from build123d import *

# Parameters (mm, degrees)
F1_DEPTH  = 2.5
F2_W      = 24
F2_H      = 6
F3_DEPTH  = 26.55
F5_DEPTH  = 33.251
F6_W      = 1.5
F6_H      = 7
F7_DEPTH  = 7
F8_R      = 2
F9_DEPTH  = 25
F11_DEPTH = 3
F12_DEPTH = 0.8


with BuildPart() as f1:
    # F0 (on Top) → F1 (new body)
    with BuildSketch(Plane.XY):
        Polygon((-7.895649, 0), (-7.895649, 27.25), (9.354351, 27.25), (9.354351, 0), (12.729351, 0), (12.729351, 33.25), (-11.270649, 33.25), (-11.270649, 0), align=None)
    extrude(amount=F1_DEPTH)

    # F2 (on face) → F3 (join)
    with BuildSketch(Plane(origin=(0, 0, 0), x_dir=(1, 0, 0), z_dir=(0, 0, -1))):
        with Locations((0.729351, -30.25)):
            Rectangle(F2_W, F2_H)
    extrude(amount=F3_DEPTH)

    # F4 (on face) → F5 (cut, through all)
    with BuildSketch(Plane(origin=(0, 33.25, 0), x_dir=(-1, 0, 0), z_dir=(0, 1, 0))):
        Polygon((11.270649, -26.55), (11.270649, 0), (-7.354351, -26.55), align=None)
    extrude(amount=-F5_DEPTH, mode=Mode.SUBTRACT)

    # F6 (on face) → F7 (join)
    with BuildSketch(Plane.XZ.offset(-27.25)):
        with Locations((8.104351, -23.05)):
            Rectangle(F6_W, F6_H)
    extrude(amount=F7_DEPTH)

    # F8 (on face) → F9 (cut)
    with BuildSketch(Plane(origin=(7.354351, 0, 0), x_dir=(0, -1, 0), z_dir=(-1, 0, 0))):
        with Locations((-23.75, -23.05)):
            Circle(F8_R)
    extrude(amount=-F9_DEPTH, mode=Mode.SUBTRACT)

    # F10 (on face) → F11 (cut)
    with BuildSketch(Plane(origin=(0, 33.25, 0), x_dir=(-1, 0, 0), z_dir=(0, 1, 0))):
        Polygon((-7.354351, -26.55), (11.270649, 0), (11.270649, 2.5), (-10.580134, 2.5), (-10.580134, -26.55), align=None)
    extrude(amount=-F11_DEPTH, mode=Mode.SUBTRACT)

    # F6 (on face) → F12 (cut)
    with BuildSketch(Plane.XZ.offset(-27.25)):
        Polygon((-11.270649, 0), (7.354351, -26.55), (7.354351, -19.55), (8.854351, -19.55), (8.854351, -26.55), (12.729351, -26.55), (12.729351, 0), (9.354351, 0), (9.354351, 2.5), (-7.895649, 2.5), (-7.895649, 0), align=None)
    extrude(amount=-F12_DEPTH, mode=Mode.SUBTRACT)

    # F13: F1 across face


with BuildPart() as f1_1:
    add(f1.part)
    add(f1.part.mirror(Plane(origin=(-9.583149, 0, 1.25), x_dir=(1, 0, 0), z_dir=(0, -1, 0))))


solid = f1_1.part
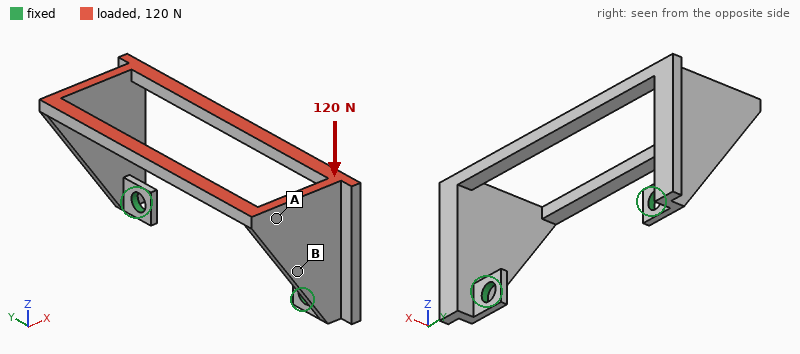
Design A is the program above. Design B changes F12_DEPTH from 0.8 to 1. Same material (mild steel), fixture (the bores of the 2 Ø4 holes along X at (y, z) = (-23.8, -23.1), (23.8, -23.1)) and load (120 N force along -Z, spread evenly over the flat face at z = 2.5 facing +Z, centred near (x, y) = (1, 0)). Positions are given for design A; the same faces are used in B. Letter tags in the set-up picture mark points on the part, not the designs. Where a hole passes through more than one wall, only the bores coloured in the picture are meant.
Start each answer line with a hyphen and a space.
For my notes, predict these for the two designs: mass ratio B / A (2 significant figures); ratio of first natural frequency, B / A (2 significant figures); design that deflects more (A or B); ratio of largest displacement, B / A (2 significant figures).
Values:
- 0.95
- 0.97
- B
- 1.1
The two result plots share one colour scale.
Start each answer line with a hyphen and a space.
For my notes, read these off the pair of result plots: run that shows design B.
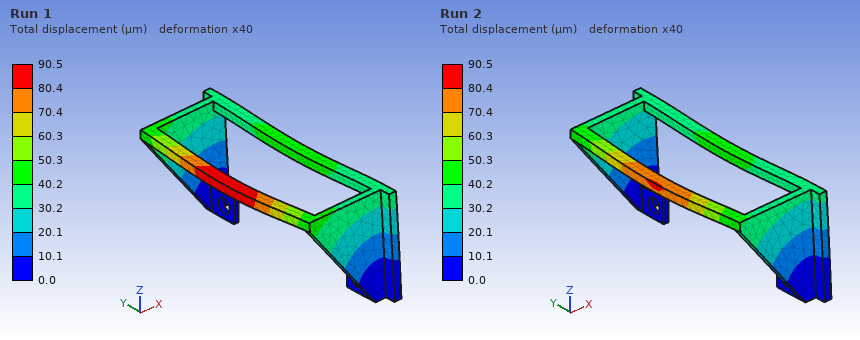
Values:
- Run 1
